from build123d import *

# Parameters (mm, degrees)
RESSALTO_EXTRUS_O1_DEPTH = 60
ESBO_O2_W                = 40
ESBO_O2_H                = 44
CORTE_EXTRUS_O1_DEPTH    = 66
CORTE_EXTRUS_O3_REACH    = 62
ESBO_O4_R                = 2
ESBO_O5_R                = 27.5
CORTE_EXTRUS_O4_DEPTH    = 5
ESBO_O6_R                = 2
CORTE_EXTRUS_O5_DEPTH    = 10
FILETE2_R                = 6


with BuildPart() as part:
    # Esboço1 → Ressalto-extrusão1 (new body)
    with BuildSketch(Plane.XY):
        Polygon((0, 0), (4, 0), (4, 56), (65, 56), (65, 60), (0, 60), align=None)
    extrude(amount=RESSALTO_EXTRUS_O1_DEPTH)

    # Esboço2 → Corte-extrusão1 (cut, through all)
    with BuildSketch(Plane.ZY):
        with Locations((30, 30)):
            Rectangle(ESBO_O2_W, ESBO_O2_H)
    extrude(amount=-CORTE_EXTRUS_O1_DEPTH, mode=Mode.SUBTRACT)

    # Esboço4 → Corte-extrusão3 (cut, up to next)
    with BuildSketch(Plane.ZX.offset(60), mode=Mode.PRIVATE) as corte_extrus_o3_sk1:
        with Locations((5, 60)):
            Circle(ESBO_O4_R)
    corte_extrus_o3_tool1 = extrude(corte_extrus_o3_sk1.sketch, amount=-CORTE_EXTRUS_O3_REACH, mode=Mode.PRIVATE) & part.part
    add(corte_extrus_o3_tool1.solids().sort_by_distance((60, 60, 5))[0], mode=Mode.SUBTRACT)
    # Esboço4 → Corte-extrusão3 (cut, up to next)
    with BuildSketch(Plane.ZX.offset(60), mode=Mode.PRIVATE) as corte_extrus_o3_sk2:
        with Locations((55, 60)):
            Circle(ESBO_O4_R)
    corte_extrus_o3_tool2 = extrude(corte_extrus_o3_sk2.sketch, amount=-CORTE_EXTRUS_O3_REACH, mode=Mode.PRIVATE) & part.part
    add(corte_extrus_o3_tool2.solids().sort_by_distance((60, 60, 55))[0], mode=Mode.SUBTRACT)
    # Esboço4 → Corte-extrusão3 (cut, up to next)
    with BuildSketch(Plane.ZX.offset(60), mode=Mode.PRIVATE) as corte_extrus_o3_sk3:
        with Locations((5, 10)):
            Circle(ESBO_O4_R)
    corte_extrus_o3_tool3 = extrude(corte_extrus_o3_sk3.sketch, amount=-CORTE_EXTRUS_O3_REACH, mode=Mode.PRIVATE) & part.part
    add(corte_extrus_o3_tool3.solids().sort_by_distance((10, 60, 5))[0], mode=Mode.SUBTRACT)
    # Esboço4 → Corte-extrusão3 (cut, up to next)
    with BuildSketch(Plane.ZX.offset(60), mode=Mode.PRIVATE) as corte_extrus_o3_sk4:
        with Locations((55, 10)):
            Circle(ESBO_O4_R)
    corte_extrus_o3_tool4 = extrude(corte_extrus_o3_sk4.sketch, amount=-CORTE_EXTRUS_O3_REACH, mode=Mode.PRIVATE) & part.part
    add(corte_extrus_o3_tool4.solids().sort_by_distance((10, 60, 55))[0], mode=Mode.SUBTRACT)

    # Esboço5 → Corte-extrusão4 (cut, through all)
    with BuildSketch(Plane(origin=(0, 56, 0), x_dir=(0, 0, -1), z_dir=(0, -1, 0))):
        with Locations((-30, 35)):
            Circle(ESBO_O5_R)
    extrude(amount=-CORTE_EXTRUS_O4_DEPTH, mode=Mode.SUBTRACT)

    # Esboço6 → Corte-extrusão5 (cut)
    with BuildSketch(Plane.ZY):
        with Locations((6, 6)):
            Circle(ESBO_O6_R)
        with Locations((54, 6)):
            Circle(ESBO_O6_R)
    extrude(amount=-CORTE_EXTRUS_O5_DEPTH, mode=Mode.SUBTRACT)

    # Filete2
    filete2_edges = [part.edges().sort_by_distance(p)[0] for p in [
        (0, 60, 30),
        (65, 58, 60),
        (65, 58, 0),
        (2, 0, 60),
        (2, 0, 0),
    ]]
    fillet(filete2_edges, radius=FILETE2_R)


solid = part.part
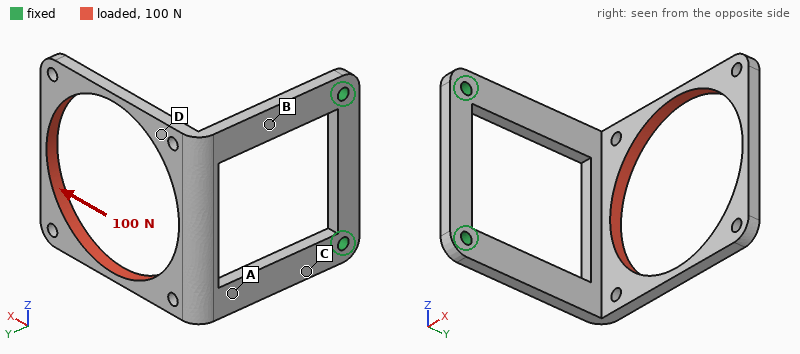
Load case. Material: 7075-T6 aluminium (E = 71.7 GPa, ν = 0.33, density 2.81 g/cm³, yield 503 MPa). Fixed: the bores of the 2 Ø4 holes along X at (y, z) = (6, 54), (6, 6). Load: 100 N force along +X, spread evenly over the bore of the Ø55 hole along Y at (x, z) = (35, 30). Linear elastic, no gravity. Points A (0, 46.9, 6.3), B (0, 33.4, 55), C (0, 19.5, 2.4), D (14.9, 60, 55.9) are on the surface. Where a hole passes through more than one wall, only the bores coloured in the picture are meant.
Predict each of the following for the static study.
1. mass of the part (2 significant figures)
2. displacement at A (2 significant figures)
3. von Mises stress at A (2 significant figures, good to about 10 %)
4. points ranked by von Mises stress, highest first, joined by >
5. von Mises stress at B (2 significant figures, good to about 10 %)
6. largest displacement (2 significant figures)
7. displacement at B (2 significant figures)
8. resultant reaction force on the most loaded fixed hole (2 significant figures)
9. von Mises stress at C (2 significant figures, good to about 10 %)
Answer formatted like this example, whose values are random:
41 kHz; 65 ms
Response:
33 g; 0.39 mm; 21 MPa; C > B > A > D; 46 MPa; 1.2 mm; 0.19 mm; 50 N; 72 MPa
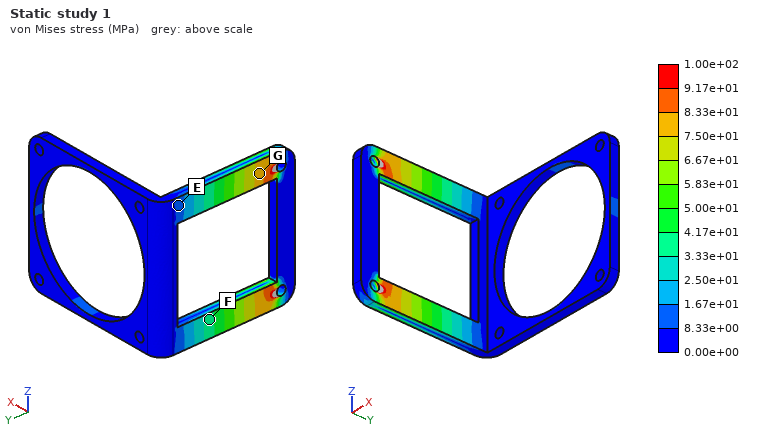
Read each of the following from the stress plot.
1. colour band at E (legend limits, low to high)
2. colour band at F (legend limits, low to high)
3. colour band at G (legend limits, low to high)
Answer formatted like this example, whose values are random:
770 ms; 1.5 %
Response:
8.33e+00 to 1.67e+01 MPa; 3.33e+01 to 4.17e+01 MPa; 7.50e+01 to 8.33e+01 MPa
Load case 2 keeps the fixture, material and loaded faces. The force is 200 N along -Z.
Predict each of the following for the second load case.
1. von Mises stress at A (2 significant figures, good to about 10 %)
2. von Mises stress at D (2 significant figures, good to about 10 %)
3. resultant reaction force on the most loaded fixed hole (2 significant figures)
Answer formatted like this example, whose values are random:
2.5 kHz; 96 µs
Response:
52 MPa; 16 MPa; 170 N
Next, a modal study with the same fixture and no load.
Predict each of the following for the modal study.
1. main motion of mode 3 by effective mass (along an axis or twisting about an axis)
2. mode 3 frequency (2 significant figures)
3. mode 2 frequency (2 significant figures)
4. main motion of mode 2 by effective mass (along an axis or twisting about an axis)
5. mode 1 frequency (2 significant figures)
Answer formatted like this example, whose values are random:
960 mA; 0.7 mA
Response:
along X; 760 Hz; 560 Hz; along Z; 310 Hz
